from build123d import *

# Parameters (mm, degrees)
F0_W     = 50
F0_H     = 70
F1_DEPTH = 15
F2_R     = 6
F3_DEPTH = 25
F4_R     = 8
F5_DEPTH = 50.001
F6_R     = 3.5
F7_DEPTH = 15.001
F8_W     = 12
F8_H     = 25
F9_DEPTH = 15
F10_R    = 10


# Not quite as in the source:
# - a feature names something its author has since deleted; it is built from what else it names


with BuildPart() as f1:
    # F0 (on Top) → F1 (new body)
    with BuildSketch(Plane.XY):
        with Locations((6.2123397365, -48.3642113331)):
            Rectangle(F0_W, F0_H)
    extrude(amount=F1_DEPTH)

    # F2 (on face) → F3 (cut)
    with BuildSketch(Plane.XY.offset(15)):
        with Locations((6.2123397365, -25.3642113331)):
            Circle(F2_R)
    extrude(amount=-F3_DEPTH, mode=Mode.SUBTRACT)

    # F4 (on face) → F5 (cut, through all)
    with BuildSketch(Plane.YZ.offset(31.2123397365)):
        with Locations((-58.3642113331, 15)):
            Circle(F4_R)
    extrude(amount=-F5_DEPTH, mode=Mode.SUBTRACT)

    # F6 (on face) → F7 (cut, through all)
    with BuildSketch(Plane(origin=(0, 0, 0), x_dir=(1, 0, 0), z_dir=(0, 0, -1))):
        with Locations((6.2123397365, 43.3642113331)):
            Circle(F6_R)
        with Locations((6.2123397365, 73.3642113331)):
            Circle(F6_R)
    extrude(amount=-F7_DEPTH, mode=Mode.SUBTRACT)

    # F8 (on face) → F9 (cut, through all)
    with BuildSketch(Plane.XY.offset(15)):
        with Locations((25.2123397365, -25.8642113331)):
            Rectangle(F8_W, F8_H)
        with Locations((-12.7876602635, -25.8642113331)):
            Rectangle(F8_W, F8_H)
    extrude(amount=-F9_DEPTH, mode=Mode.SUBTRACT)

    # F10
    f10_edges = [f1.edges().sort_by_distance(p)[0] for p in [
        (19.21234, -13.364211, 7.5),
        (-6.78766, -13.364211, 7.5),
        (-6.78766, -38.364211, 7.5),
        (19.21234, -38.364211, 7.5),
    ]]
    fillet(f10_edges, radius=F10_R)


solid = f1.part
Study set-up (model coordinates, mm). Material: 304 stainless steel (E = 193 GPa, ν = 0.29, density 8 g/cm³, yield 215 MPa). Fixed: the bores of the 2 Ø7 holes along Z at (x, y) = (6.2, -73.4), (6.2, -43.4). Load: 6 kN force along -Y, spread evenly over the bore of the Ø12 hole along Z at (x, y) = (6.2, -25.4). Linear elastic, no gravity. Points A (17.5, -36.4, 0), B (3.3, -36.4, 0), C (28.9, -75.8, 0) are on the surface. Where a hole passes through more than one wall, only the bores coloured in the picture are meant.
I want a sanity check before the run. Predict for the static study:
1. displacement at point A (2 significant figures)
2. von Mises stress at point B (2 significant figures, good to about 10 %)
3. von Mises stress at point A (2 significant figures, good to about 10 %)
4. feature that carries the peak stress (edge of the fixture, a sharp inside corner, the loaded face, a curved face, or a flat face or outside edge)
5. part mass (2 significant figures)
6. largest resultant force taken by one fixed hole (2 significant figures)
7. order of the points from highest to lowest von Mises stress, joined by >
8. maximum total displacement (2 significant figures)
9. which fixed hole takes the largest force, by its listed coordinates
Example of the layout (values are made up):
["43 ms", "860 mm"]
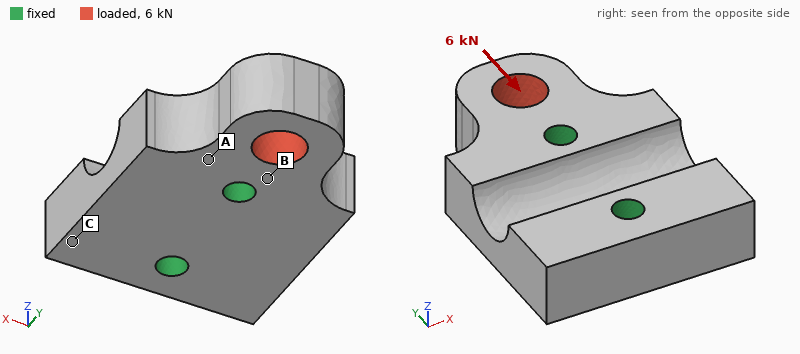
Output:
["1.1 µm", "19 MPa", "11 MPa", "the loaded face", "280 g", "5.1 kN", "B > A > C", "3.8 µm", "(6.2, -43.4)"]
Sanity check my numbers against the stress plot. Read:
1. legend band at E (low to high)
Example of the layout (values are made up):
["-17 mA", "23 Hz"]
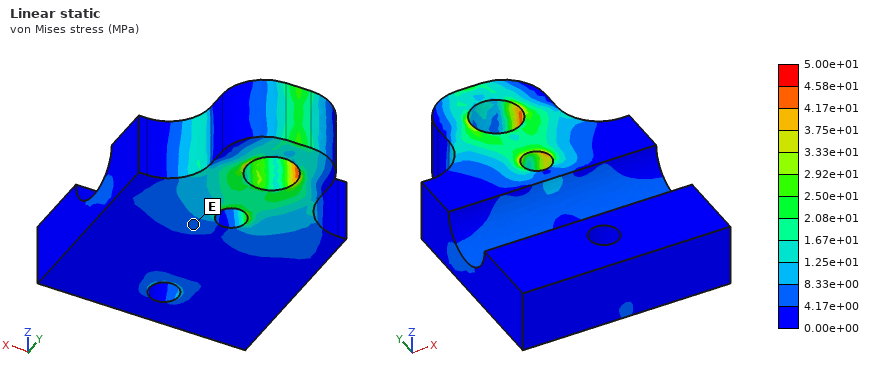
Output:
["4.17e+00 to 8.33e+00 MPa"]
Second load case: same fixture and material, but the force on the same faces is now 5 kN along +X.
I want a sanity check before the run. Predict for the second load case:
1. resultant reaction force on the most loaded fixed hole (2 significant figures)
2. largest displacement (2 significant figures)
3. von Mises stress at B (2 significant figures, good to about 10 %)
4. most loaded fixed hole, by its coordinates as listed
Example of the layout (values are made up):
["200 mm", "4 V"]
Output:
["6.8 kN", "13 µm", "32 MPa", "(6.2, -43.4)"]
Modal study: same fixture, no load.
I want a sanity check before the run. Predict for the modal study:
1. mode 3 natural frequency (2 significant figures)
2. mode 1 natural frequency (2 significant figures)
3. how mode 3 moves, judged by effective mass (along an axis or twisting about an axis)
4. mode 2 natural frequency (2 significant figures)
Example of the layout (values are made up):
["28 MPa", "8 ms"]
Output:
["15 kHz", "13 kHz", "twisting about Y", "14 kHz"]
